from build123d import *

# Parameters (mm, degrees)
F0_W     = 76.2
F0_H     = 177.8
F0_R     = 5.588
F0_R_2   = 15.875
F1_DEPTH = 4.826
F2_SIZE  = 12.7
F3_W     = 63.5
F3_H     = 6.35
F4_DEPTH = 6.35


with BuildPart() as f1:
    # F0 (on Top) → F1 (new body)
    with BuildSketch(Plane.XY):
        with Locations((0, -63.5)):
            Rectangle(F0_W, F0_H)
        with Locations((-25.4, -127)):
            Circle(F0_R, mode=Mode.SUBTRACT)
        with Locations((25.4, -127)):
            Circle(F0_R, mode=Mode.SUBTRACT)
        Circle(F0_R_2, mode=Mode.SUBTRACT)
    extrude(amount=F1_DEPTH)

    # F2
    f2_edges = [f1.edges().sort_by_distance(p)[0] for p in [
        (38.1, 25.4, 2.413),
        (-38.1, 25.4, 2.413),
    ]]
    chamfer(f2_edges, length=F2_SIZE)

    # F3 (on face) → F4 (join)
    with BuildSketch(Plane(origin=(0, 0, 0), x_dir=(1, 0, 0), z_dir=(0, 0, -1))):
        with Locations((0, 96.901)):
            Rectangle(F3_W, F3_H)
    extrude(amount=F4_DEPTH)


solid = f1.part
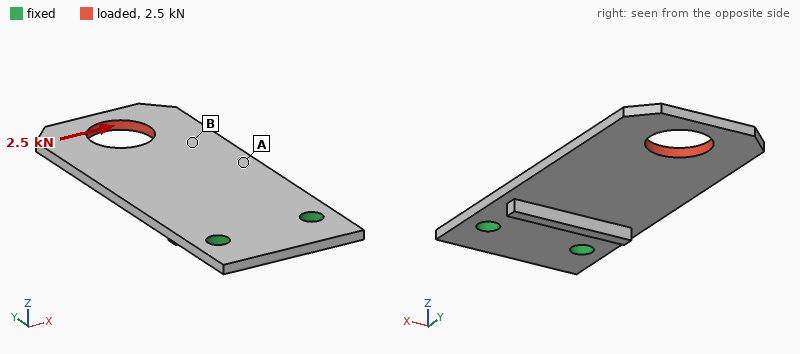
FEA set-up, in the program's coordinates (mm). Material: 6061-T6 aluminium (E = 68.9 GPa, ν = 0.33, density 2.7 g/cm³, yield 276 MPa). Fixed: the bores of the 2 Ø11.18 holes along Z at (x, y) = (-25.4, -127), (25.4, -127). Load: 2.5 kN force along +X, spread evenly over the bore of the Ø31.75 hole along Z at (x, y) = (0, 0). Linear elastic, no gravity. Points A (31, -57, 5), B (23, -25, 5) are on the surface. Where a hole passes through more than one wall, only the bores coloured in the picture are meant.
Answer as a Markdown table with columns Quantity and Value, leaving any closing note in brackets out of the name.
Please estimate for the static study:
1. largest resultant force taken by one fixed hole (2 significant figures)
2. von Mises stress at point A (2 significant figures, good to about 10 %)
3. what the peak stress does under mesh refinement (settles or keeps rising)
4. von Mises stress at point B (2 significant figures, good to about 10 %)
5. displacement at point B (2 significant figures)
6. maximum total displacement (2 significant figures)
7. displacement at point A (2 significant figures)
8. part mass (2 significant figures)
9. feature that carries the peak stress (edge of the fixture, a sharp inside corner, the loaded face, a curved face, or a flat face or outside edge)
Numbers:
| Quantity | Value |
|---|---|
| largest resultant force taken by one fixed hole | 5.8 kN |
| von Mises stress at point A | 26 MPa |
| what the peak stress does under mesh refinement | keeps rising |
| von Mises stress at point B | 9.4 MPa |
| displacement at point B | 0.13 mm |
| maximum total displacement | 0.24 mm |
| displacement at point A | 0.083 mm |
| part mass | 170 g |
| feature that carries the peak stress | edge of the fixture |
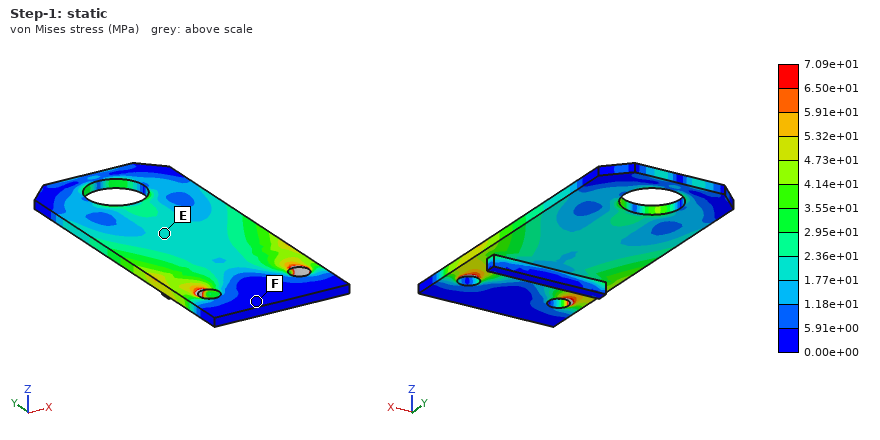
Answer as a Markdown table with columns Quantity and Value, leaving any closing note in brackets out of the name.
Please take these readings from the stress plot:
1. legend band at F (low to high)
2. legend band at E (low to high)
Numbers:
| Quantity | Value |
|---|---|
| legend band at F | 0.00e+00 to 5.91e+00 MPa |
| legend band at E | 1.77e+01 to 2.36e+01 MPa |
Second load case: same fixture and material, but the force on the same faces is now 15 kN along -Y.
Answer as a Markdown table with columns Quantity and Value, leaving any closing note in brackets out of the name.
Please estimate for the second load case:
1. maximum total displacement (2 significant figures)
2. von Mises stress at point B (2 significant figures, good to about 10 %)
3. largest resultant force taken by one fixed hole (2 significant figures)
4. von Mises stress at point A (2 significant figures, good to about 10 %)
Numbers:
| Quantity | Value |
|---|---|
| maximum total displacement | 0.15 mm |
| von Mises stress at point B | 52 MPa |
| largest resultant force taken by one fixed hole | 7.6 kN |
| von Mises stress at point A | 43 MPa |
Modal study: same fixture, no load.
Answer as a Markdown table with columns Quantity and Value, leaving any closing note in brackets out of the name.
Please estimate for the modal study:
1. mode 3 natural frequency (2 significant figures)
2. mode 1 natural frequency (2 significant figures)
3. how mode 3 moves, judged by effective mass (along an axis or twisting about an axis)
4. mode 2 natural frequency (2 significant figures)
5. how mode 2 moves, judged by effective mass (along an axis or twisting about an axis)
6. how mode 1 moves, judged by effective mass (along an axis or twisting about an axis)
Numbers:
| Quantity | Value |
|---|---|
| mode 3 natural frequency | 1100 Hz |
| mode 1 natural frequency | 210 Hz |
| how mode 3 moves, judged by effective mass | along Z |
| mode 2 natural frequency | 800 Hz |
| how mode 2 moves, judged by effective mass | twisting about Y |
| how mode 1 moves, judged by effective mass | along Z |
